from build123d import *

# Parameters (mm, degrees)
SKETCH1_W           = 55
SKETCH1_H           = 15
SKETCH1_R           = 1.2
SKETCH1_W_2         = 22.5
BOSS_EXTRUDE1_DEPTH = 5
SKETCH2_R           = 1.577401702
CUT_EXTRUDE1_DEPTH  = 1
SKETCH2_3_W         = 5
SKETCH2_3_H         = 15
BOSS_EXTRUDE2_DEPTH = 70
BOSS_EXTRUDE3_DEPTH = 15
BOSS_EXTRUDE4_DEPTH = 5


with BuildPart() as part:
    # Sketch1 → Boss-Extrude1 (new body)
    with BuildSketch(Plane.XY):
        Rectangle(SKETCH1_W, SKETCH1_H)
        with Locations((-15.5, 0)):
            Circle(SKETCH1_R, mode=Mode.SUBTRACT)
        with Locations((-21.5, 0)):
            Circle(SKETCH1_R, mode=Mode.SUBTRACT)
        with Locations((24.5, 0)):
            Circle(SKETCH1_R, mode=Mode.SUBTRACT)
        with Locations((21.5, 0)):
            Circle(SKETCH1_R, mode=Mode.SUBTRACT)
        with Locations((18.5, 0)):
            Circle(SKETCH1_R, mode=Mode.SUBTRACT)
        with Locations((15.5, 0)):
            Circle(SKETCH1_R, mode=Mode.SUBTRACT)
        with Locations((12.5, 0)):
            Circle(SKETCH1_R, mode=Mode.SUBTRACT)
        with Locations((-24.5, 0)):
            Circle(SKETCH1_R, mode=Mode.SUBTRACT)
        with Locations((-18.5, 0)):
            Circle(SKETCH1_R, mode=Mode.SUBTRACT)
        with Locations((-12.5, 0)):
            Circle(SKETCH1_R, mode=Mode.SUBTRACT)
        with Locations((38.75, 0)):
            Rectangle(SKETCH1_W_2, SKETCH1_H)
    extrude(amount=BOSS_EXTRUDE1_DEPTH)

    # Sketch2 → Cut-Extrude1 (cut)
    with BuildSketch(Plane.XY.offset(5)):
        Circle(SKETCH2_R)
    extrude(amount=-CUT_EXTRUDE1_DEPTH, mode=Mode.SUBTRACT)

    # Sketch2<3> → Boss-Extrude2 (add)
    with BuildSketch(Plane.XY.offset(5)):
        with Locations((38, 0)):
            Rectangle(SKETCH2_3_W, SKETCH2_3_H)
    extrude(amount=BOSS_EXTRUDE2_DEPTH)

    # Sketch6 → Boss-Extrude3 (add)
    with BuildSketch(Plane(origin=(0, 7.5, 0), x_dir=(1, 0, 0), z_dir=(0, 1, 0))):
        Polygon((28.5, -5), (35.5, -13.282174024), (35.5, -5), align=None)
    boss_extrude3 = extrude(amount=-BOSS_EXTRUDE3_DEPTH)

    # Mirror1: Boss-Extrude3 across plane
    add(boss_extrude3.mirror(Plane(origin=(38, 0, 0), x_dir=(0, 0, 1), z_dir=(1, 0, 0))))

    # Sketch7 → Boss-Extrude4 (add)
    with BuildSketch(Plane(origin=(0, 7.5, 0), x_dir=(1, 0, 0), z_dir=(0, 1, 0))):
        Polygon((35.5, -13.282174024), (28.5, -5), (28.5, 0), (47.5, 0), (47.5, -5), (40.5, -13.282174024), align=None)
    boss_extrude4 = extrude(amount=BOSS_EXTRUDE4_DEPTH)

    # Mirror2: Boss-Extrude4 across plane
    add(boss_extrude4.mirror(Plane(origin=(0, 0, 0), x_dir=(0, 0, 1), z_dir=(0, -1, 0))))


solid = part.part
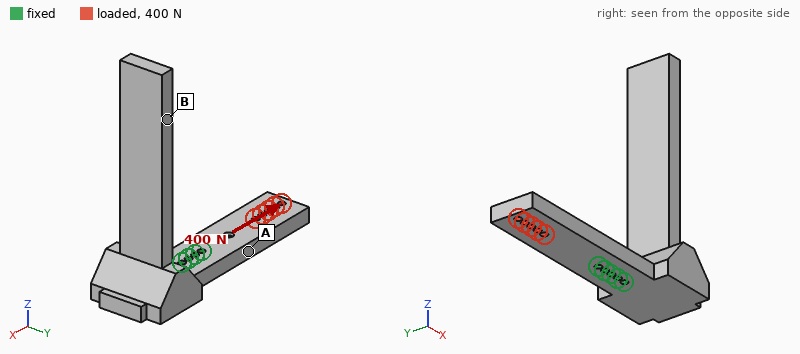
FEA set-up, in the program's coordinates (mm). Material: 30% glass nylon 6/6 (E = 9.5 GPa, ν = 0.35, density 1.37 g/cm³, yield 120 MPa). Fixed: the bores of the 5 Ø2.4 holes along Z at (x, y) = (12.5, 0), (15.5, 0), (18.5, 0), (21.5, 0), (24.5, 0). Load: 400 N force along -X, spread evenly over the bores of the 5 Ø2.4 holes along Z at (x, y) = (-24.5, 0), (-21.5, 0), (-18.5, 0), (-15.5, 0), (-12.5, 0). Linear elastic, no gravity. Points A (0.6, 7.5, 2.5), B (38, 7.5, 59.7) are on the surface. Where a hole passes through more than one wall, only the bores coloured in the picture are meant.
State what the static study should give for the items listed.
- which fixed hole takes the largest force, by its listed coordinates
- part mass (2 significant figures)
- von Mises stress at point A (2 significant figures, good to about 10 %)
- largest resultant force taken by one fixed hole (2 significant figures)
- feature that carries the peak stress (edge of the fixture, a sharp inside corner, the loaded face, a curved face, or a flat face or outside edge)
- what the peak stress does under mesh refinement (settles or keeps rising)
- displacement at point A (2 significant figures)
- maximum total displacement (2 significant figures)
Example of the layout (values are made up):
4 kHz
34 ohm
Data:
(12.5, 0)
19 g
5.2 MPa
250 N
edge of the fixture
keeps rising
8.6 µm
24 µm
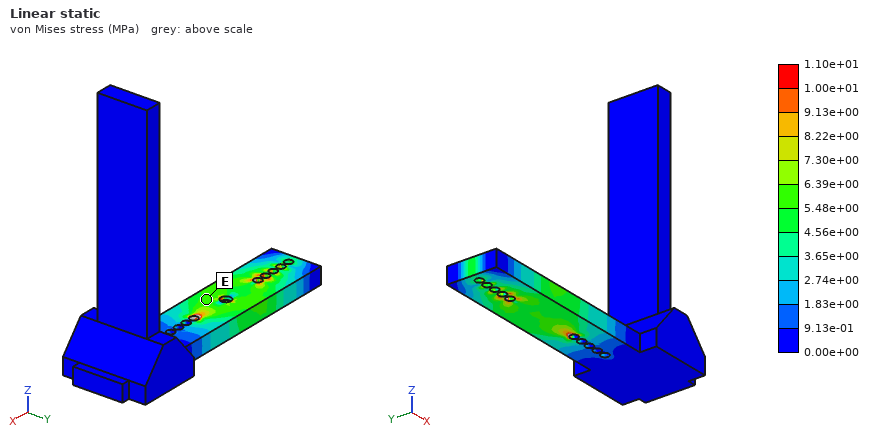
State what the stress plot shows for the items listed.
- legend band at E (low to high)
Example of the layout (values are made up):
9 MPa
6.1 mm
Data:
5.48e+00 to 6.39e+00 MPa
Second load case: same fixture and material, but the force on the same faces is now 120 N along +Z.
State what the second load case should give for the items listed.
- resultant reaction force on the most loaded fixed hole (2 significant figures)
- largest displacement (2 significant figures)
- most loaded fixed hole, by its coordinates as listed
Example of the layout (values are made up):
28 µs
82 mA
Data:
350 N
1.3 mm
(12.5, 0)
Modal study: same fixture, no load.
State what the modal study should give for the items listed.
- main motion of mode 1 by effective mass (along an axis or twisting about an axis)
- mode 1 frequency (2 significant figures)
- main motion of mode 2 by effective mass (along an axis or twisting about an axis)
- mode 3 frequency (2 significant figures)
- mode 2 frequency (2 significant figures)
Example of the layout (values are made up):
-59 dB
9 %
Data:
along X
410 Hz
along Y
1300 Hz
680 Hz
